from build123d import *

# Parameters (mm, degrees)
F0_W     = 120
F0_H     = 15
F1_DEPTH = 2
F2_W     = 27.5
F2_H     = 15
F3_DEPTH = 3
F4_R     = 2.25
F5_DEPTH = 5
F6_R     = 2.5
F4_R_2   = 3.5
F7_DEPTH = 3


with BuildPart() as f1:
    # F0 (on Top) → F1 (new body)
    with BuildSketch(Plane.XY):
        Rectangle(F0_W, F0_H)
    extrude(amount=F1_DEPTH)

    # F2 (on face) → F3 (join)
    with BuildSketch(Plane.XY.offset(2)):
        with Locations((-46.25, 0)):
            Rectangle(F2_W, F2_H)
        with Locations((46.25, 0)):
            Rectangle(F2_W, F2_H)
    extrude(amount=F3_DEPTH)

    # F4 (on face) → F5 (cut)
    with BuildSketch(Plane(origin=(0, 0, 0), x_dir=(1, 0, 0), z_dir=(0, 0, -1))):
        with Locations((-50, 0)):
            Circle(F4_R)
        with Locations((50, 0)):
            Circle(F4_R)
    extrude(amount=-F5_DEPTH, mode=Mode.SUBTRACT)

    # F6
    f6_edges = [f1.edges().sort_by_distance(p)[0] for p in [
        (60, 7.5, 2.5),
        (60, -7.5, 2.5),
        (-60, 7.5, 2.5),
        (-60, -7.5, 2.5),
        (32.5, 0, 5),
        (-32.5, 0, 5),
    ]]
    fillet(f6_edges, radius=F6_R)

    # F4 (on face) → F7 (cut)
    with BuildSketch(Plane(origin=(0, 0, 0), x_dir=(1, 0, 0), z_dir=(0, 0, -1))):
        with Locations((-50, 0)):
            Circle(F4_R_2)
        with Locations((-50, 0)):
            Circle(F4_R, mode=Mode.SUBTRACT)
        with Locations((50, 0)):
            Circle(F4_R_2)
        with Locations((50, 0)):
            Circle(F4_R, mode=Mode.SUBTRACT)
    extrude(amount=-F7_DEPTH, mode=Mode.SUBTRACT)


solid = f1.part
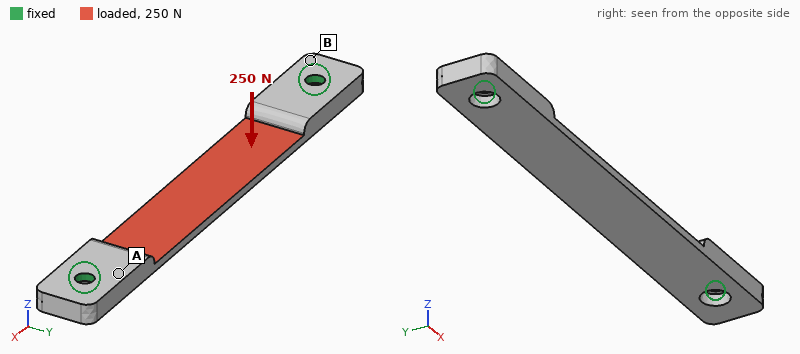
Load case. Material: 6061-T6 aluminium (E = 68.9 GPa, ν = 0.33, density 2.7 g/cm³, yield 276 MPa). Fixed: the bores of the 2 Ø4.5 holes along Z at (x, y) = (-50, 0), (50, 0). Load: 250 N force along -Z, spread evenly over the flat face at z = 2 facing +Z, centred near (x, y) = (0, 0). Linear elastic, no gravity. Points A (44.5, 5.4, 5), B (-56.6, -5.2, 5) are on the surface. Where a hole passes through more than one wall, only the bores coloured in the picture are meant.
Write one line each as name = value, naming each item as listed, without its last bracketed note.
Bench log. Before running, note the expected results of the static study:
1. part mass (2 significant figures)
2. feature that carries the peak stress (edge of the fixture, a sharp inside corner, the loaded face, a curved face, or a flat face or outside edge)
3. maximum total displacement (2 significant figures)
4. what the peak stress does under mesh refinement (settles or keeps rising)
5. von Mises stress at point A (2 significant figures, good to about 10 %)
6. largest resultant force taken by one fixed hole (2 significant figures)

part mass = 15 g
feature that carries the peak stress = edge of the fixture
maximum total displacement = 0.40 mm
what the peak stress does under mesh refinement = keeps rising
von Mises stress at point A = 37 MPa
largest resultant force taken by one fixed hole = 450 N
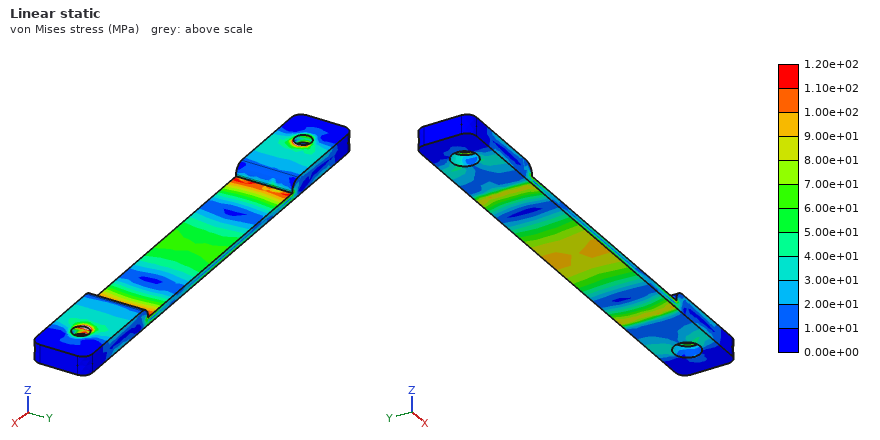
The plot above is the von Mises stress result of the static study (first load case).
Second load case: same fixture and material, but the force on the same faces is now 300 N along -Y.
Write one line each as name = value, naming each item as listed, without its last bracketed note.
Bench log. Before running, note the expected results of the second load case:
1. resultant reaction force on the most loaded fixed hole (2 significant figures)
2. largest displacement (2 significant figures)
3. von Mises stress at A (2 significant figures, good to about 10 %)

resultant reaction force on the most loaded fixed hole = 150 N
largest displacement = 48 µm
von Mises stress at A = 8.8 MPa
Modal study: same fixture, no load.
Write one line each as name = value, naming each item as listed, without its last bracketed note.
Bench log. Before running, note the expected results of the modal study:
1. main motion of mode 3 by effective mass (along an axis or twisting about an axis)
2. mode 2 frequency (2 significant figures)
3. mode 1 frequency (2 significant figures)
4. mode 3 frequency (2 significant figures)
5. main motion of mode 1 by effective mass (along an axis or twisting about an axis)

main motion of mode 3 by effective mass = along Y
mode 2 frequency = 4200 Hz
mode 1 frequency = 2000 Hz
mode 3 frequency = 5800 Hz
main motion of mode 1 by effective mass = along Z
